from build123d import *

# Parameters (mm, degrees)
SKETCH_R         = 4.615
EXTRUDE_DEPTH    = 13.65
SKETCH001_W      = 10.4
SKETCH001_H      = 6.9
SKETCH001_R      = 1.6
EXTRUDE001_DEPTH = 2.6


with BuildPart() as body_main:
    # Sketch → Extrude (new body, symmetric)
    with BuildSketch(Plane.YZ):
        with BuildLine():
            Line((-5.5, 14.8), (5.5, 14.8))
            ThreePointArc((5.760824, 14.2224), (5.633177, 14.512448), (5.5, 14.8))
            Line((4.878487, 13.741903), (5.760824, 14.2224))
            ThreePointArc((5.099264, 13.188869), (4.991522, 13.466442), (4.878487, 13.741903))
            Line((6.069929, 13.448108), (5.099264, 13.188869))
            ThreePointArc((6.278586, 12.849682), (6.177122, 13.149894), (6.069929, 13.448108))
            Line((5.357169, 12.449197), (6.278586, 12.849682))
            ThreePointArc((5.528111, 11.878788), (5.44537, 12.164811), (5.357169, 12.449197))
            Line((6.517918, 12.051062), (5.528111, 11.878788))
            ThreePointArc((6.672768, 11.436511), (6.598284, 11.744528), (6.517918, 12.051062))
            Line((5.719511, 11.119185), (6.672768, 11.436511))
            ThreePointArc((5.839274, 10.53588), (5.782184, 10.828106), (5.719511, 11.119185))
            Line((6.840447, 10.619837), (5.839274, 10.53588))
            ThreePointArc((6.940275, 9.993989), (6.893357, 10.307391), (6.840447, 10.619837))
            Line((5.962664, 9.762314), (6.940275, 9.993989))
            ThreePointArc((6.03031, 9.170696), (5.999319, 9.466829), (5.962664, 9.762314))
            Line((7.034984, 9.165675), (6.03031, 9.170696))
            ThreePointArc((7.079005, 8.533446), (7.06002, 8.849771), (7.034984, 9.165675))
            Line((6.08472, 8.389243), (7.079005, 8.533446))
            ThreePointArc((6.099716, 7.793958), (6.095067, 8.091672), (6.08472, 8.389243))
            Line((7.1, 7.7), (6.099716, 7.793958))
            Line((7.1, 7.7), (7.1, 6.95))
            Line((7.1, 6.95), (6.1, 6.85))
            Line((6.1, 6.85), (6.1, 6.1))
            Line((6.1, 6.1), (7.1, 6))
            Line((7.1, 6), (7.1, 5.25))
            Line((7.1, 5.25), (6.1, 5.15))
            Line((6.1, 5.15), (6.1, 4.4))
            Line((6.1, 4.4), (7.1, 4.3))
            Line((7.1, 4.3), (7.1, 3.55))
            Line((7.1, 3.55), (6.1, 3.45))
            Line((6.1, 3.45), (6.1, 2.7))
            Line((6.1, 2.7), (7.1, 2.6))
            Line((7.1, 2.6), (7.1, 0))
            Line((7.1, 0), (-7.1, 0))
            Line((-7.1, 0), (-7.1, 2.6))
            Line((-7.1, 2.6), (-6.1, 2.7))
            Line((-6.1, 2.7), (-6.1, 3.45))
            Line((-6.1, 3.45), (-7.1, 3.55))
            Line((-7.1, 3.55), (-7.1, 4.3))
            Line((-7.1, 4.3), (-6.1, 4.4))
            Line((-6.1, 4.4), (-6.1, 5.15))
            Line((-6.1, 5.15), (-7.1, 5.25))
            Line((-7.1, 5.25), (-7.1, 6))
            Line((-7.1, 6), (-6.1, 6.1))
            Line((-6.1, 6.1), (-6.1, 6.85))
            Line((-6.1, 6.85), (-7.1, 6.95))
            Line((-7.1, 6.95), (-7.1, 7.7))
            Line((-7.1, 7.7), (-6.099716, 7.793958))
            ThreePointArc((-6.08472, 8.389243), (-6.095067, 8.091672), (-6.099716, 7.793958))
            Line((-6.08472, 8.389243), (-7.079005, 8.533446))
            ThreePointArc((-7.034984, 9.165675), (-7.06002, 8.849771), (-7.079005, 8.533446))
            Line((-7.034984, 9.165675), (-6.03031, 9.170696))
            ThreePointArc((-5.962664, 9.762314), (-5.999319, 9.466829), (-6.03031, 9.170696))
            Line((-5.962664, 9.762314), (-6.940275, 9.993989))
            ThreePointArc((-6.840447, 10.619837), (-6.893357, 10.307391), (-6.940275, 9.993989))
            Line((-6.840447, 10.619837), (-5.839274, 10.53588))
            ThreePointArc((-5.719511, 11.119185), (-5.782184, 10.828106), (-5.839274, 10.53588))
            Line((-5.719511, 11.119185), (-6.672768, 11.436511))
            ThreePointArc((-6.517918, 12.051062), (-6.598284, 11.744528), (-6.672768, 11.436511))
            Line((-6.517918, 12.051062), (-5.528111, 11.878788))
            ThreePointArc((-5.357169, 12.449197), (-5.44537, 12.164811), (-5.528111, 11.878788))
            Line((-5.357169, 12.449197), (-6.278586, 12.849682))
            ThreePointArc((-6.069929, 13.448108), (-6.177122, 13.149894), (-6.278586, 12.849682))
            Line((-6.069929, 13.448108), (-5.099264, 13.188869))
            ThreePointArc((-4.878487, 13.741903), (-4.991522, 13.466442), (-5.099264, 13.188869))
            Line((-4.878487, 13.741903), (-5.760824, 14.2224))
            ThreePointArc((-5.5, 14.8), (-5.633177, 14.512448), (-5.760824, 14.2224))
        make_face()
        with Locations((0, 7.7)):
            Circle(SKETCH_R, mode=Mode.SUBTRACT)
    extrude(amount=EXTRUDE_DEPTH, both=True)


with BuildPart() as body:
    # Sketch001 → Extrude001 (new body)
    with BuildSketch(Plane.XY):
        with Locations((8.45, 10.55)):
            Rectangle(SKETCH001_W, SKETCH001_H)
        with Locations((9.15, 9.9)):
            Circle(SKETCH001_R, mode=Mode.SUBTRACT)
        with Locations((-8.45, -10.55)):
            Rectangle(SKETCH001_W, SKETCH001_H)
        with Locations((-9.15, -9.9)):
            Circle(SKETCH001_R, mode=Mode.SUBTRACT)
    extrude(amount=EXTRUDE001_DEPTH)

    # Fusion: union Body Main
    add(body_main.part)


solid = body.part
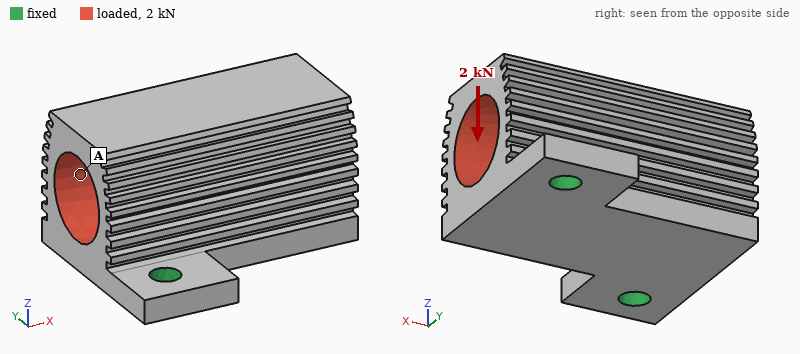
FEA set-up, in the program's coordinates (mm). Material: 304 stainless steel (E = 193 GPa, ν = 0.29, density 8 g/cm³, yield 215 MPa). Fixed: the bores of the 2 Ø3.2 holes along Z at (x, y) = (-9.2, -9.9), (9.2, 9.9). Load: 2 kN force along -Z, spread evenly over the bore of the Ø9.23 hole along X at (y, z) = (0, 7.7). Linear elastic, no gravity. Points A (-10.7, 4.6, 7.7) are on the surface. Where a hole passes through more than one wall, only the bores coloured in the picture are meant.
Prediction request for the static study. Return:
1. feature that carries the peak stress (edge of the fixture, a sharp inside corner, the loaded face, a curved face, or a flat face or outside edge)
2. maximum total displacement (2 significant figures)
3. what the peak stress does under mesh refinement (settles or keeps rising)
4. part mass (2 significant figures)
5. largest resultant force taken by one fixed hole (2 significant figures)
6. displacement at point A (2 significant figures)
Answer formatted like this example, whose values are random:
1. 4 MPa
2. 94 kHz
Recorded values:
1. edge of the fixture
2. 11 µm
3. keeps rising
4. 30 g
5. 1.0 kN
6. 10 µm
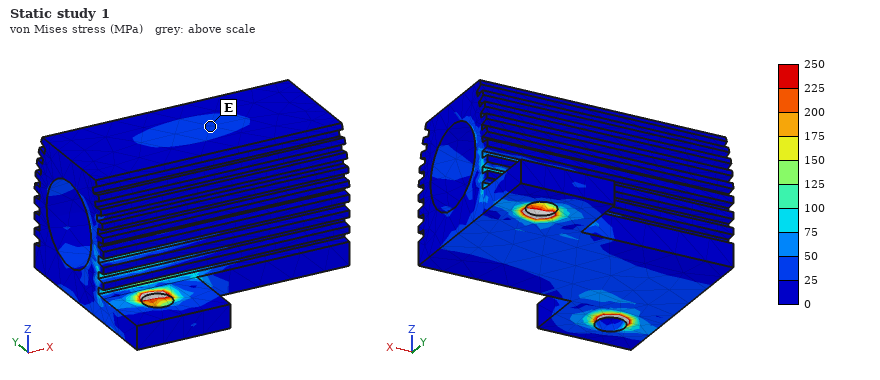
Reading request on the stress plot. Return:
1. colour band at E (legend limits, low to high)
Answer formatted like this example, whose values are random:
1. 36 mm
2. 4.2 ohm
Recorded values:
1. 25 to 50 MPa
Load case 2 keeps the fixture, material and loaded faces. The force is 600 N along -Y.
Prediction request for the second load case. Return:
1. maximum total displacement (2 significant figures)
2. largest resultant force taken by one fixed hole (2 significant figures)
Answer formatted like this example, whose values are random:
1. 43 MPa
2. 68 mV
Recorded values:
1. 29 µm
2. 330 N
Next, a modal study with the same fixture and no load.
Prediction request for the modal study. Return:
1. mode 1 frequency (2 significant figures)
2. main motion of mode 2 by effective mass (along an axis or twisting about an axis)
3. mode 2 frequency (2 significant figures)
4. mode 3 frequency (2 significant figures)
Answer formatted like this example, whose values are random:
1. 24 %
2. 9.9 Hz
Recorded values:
1. 4500 Hz
2. along Z
3. 15 kHz
4. 16 kHz
